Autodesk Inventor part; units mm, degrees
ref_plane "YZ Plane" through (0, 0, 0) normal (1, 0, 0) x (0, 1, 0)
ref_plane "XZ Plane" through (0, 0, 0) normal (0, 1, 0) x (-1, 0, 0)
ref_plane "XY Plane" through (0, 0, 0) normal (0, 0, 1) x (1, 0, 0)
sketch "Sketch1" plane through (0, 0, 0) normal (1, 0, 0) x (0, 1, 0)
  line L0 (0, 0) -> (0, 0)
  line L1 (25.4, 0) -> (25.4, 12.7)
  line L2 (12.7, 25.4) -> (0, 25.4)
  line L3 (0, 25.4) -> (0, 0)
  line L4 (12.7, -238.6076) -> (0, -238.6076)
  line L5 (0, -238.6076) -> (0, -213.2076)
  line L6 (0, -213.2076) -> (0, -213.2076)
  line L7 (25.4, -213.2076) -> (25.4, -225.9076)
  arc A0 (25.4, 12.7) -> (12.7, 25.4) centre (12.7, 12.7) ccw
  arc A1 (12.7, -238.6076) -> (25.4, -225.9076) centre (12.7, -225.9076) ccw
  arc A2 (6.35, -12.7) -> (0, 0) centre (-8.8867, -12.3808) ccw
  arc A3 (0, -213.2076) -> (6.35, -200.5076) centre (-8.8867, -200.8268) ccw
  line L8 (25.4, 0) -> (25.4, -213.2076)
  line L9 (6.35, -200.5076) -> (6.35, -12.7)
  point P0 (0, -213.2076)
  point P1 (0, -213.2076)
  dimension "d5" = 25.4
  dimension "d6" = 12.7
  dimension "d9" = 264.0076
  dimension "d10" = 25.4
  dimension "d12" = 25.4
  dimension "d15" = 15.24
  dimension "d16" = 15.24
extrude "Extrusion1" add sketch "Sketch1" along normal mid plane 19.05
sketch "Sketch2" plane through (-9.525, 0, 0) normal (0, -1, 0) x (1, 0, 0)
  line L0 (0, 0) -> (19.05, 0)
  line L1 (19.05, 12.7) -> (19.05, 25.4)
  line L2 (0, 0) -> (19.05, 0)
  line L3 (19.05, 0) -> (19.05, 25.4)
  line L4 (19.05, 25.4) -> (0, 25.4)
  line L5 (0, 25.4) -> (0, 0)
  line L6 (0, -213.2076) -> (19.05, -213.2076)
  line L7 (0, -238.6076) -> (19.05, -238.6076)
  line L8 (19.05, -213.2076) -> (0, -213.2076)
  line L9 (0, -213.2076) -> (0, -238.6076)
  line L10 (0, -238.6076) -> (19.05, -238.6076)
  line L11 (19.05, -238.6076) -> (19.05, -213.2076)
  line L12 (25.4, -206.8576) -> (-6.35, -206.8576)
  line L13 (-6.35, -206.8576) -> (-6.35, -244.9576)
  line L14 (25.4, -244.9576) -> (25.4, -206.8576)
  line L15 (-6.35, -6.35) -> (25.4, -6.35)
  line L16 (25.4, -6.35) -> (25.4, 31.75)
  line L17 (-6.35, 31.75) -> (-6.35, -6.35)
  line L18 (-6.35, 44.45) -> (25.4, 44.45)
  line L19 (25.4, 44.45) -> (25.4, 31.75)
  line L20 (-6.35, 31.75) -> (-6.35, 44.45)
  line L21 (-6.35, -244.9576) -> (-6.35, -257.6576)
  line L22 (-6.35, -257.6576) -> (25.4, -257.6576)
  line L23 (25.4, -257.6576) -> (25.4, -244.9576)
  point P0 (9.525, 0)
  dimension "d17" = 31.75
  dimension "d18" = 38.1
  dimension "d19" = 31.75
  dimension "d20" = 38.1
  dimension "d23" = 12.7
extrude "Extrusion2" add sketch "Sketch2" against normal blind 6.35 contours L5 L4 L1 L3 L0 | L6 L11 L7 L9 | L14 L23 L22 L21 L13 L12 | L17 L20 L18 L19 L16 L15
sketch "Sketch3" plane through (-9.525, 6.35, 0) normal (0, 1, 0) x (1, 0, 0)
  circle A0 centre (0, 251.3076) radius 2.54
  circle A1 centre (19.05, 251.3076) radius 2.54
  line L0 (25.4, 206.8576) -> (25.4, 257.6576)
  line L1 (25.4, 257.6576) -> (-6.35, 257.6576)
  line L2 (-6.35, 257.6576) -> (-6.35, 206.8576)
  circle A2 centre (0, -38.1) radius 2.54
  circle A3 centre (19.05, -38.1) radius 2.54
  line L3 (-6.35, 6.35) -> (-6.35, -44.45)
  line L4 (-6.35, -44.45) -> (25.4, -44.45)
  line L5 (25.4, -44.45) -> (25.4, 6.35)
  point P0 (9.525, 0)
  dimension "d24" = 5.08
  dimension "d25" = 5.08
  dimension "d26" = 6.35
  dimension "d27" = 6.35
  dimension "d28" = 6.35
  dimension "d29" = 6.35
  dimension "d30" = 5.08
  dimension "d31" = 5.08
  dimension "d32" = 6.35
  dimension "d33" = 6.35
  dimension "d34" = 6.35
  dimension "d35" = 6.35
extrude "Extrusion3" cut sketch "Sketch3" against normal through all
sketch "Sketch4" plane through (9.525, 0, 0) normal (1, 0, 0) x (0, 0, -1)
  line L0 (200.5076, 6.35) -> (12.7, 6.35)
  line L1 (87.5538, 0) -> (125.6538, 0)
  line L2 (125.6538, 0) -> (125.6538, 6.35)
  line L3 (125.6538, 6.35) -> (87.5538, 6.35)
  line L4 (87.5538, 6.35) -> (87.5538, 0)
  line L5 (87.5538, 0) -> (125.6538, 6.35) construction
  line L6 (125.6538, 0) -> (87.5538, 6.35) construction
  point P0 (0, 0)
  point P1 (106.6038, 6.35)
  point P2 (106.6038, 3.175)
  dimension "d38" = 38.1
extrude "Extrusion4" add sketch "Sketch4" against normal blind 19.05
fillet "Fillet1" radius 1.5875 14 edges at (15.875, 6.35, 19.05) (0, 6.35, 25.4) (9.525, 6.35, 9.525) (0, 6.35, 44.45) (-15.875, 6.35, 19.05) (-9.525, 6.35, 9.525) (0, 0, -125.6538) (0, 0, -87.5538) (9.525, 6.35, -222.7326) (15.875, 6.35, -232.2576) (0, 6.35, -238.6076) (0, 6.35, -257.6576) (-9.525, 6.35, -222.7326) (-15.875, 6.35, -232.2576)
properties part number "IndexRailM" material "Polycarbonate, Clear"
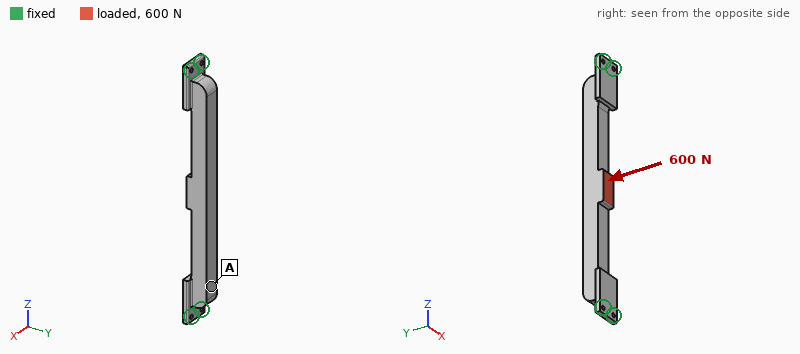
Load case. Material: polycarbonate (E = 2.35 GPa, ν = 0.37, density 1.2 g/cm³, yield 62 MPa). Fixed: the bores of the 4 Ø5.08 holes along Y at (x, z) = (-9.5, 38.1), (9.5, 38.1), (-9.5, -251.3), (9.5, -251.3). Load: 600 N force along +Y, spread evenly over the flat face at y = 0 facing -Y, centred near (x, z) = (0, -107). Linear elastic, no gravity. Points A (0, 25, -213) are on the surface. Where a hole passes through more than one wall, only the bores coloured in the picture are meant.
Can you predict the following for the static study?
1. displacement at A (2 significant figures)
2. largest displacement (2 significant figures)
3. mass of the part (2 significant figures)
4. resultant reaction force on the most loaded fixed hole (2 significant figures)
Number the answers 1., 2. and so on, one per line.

1. 0.77 mm
2. 2.8 mm
3. 140 g
4. 690 N
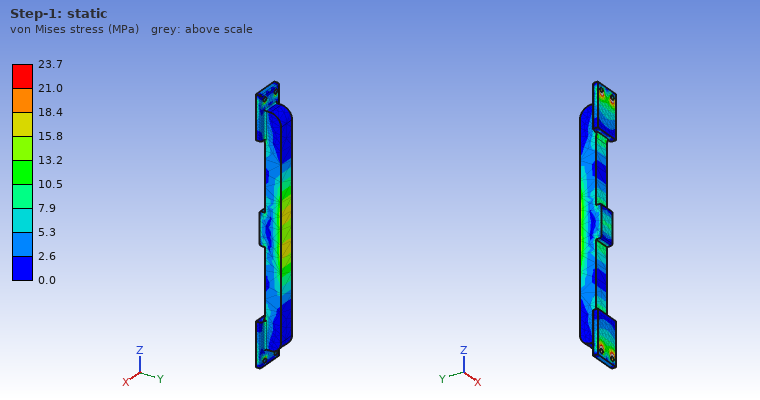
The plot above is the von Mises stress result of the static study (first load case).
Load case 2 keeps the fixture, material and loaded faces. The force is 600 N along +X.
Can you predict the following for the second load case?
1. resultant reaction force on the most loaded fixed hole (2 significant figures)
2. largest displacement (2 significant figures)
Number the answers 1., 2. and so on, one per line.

1. 1.1 kN
2. 3.0 mm
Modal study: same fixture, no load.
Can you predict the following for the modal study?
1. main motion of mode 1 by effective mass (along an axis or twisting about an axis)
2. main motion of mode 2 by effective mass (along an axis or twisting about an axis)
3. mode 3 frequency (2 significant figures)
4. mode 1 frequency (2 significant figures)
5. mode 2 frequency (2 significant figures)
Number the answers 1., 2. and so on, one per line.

1. along Y
2. along X
3. 600 Hz
4. 300 Hz
5. 330 Hz
